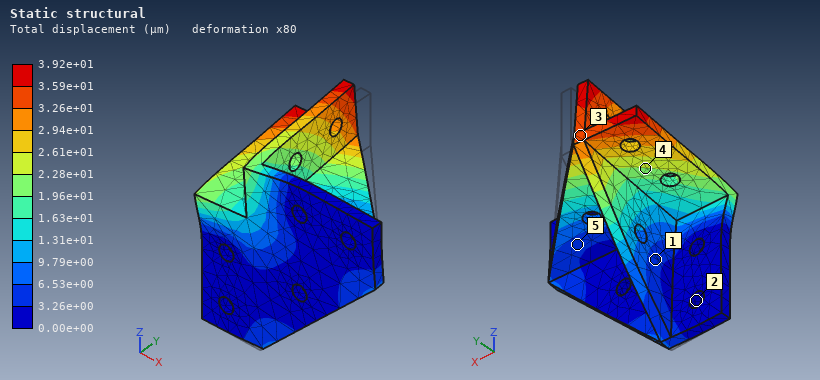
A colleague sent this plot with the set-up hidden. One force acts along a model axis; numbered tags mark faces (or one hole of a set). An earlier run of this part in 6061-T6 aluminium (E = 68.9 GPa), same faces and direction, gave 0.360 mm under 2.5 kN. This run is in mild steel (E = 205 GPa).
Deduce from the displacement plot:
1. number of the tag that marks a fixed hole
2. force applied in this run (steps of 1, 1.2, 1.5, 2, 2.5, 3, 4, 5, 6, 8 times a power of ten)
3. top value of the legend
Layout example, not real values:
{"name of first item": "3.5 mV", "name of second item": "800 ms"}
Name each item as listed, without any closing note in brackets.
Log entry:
{"number of the tag that marks a fixed hole": "2", "force applied in this run": "800 N", "top value of the legend": "3.92e+01 µm"}
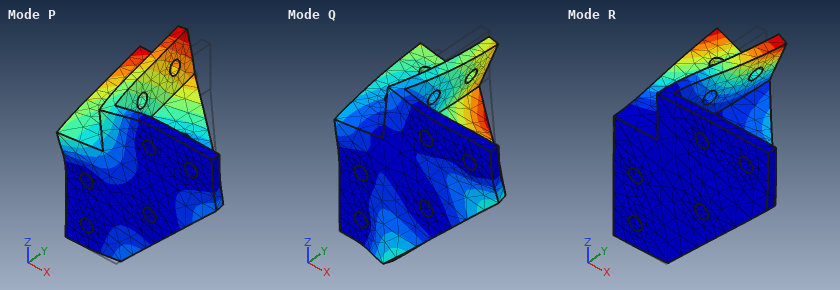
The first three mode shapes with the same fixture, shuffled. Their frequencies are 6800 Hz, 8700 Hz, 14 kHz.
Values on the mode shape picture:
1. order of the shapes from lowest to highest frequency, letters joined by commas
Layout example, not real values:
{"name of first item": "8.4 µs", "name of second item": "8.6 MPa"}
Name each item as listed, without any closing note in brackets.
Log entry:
{"order of the shapes from lowest to highest frequency, letters joined by commas": "P, R, Q"}
